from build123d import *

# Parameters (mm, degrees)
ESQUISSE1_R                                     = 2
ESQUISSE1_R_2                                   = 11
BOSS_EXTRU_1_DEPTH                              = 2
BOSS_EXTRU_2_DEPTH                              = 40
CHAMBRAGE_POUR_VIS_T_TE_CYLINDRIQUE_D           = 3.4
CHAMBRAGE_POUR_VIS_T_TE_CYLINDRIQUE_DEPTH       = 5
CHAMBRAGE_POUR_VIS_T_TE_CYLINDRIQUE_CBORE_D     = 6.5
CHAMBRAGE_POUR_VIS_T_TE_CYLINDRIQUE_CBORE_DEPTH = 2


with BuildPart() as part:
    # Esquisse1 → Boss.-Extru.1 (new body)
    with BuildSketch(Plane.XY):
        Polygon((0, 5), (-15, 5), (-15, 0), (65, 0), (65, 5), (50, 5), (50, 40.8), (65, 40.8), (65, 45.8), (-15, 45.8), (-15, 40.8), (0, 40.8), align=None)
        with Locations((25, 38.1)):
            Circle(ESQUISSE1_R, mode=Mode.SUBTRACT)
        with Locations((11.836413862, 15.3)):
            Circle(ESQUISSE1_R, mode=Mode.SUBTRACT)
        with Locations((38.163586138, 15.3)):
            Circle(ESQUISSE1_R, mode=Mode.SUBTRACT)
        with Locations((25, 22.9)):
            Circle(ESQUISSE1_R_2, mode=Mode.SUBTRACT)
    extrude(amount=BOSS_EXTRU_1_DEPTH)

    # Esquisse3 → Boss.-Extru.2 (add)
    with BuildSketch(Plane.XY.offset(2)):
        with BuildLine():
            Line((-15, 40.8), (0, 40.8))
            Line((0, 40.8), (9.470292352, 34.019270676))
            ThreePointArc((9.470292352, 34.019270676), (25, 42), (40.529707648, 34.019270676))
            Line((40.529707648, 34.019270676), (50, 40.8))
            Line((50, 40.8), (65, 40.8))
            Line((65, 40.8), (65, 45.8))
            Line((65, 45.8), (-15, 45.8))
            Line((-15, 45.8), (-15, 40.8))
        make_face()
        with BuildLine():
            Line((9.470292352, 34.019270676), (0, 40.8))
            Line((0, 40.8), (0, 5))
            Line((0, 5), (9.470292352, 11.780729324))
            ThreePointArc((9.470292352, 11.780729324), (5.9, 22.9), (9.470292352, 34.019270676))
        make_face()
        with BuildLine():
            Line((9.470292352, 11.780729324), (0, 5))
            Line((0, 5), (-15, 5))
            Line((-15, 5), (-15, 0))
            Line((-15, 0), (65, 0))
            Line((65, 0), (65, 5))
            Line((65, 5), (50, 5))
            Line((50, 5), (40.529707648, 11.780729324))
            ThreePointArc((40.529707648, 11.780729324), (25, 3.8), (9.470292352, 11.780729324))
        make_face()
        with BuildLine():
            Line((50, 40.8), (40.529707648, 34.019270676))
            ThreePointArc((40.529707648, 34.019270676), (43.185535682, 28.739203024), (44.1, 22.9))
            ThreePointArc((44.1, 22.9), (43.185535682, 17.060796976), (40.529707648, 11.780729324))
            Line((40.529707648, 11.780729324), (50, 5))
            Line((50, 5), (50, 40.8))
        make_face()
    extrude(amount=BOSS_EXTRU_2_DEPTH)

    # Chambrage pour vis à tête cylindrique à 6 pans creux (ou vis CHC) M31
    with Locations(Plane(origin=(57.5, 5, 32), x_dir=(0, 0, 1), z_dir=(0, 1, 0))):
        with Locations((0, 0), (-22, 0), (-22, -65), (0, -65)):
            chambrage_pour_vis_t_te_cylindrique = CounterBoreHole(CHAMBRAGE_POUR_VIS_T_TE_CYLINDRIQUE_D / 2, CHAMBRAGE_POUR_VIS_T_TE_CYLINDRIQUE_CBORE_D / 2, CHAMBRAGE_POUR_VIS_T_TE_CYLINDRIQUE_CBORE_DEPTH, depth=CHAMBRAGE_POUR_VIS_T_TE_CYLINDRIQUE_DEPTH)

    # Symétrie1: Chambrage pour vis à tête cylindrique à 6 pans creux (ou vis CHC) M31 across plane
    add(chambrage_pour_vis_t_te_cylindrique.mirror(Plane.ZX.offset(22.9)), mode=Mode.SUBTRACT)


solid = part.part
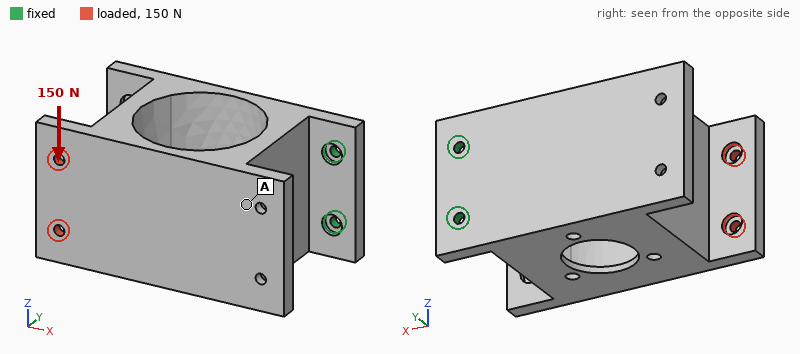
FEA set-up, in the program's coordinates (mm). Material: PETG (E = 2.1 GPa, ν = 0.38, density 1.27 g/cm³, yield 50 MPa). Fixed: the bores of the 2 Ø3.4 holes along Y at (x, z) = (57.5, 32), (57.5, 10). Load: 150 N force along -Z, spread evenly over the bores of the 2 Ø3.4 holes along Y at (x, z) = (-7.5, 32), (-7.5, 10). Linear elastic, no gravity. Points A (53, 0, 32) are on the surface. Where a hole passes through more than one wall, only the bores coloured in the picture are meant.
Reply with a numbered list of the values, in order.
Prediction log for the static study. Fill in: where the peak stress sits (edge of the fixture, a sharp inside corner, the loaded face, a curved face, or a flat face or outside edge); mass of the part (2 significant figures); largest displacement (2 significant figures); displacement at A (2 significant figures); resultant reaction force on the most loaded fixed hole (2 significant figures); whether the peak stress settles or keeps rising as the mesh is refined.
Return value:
1. edge of the fixture
2. 78 g
3. 1.2 mm
4. 0.51 mm
5. 500 N
6. keeps rising
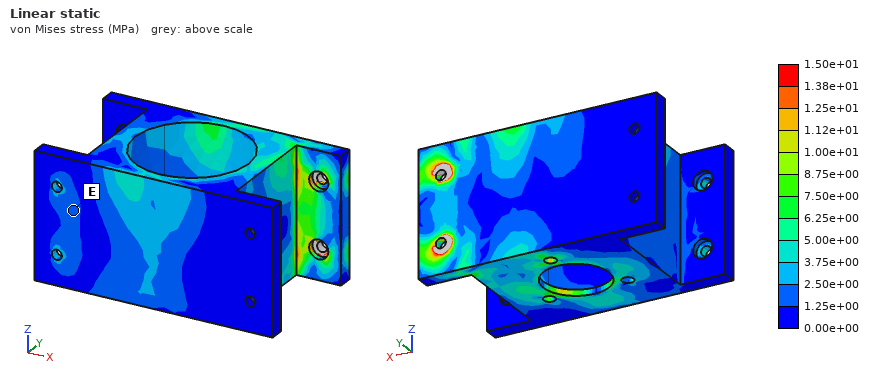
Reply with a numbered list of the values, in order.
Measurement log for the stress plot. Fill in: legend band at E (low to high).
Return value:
1. 1.25e+00 to 2.50e+00 MPa
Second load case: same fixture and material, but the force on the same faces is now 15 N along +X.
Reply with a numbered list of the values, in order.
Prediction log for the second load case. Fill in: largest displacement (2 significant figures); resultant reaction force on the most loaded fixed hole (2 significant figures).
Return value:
1. 1.0 mm
2. 7.6 N
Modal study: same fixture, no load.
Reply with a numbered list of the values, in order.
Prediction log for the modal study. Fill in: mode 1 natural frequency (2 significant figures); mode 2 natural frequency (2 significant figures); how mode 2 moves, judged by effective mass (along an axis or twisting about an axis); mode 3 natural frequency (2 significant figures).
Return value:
1. 90 Hz
2. 400 Hz
3. along Z
4. 660 Hz
